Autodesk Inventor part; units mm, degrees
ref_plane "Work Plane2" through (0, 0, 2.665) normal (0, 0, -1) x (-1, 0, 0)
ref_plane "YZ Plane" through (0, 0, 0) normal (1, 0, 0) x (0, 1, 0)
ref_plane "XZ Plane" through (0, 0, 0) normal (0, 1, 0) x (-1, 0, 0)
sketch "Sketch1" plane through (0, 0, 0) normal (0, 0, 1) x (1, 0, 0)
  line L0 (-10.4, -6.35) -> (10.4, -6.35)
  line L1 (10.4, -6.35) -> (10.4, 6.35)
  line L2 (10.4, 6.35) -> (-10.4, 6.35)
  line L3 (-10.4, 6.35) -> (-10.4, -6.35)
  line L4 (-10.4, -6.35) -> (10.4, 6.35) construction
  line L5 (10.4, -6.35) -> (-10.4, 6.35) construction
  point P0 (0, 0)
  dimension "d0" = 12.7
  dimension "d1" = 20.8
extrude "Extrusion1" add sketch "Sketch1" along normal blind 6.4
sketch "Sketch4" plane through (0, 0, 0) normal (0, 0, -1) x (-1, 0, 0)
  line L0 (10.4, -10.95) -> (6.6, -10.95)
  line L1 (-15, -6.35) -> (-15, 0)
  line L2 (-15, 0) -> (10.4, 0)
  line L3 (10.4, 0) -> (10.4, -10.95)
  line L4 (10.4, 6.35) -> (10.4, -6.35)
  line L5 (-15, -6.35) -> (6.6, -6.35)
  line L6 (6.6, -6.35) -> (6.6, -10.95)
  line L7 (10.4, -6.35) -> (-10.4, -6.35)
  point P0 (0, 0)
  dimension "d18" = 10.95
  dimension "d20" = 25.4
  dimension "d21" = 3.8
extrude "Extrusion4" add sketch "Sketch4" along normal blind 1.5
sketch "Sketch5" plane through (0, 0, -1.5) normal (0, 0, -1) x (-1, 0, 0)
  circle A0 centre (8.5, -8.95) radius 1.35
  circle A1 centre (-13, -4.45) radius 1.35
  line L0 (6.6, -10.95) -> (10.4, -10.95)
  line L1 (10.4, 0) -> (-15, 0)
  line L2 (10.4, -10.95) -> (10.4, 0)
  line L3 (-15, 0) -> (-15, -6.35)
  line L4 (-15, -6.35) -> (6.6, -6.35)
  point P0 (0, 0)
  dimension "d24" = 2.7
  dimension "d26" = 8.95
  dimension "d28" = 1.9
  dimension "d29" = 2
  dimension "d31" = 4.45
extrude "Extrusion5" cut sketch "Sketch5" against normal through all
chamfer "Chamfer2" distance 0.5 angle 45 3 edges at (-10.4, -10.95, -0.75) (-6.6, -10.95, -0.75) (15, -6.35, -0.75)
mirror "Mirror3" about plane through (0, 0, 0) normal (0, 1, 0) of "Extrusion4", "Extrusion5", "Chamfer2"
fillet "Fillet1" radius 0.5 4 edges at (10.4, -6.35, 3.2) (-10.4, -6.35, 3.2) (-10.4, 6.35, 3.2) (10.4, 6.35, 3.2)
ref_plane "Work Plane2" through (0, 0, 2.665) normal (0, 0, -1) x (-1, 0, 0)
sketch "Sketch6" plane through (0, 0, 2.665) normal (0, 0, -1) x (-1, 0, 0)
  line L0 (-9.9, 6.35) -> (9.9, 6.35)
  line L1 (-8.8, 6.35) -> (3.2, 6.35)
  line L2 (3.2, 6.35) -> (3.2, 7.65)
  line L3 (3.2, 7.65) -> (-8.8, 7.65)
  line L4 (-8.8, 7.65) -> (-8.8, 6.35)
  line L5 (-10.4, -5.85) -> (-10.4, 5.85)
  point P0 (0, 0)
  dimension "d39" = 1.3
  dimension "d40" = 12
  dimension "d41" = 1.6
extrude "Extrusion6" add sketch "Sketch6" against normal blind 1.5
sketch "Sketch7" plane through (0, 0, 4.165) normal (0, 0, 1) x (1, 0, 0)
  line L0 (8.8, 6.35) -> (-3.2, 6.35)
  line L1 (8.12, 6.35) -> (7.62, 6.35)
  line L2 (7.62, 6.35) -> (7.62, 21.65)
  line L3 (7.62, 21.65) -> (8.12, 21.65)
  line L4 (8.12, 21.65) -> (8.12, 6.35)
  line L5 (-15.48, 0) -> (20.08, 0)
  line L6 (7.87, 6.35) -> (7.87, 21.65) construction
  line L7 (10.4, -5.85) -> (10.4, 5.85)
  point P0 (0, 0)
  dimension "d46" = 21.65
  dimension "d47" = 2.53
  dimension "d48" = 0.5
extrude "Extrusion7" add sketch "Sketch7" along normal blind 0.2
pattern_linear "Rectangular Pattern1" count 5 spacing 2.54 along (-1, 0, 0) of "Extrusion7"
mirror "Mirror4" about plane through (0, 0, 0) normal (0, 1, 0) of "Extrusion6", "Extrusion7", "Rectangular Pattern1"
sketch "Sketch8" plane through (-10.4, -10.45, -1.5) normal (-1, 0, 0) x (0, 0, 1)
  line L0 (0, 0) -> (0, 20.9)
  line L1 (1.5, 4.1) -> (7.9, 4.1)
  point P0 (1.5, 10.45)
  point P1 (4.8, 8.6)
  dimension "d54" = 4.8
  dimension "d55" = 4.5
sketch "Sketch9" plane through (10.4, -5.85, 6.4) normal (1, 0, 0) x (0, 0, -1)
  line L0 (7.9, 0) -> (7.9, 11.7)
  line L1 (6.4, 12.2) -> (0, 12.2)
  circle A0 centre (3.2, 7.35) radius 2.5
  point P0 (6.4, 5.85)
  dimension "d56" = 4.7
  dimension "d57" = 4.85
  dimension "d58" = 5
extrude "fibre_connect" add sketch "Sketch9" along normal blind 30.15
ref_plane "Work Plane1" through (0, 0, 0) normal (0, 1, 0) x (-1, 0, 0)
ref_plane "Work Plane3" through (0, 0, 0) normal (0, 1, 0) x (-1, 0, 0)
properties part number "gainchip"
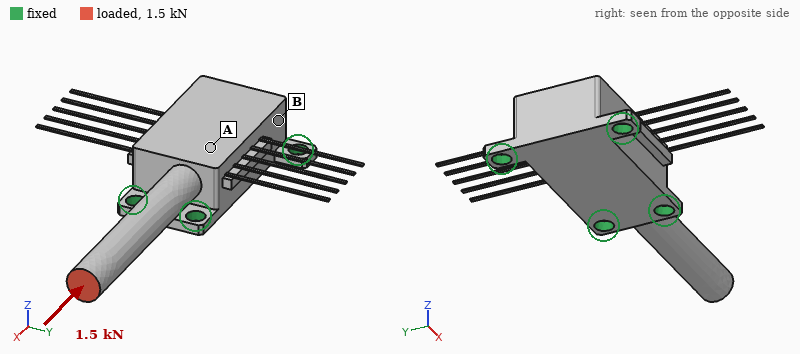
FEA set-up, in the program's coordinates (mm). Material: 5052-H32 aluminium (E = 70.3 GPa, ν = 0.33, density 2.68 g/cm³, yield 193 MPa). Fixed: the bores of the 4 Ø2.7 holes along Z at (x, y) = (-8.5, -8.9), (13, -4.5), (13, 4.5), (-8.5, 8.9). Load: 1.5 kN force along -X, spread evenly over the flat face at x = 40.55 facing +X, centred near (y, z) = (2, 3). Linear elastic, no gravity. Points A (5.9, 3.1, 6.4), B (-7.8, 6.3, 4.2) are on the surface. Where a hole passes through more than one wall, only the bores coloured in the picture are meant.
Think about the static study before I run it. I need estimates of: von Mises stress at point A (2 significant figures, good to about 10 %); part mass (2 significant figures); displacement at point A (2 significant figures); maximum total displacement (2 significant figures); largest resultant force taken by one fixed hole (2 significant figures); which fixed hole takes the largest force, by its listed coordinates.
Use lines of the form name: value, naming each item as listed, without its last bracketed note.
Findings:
von Mises stress at point A: 37 MPa
part mass: 7.6 g
displacement at point A: 9.4 µm
maximum total displacement: 55 µm
largest resultant force taken by one fixed hole: 630 N
which fixed hole takes the largest force, by its listed coordinates: (13, 4.5)
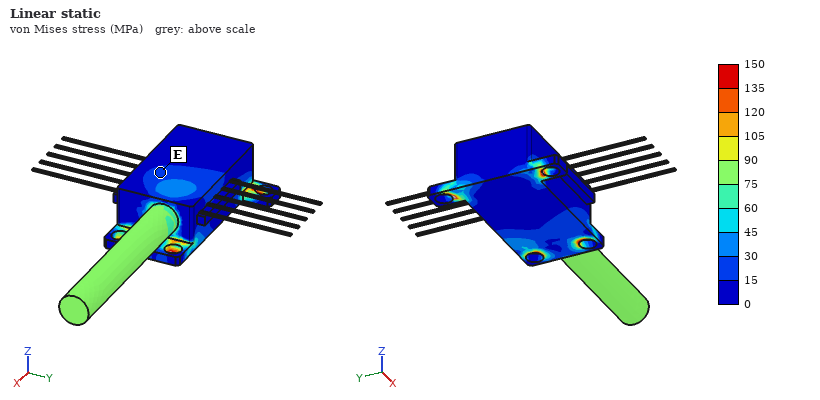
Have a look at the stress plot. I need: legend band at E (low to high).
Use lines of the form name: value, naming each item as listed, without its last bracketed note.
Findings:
legend band at E: 15 to 30 MPa
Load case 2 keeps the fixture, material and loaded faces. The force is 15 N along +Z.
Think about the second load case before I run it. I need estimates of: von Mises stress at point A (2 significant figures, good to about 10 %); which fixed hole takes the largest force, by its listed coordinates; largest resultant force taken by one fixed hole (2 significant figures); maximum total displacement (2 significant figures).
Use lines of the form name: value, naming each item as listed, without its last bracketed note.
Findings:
von Mises stress at point A: 4.9 MPa
which fixed hole takes the largest force, by its listed coordinates: (13, 4.5)
largest resultant force taken by one fixed hole: 23 N
maximum total displacement: 76 µm
